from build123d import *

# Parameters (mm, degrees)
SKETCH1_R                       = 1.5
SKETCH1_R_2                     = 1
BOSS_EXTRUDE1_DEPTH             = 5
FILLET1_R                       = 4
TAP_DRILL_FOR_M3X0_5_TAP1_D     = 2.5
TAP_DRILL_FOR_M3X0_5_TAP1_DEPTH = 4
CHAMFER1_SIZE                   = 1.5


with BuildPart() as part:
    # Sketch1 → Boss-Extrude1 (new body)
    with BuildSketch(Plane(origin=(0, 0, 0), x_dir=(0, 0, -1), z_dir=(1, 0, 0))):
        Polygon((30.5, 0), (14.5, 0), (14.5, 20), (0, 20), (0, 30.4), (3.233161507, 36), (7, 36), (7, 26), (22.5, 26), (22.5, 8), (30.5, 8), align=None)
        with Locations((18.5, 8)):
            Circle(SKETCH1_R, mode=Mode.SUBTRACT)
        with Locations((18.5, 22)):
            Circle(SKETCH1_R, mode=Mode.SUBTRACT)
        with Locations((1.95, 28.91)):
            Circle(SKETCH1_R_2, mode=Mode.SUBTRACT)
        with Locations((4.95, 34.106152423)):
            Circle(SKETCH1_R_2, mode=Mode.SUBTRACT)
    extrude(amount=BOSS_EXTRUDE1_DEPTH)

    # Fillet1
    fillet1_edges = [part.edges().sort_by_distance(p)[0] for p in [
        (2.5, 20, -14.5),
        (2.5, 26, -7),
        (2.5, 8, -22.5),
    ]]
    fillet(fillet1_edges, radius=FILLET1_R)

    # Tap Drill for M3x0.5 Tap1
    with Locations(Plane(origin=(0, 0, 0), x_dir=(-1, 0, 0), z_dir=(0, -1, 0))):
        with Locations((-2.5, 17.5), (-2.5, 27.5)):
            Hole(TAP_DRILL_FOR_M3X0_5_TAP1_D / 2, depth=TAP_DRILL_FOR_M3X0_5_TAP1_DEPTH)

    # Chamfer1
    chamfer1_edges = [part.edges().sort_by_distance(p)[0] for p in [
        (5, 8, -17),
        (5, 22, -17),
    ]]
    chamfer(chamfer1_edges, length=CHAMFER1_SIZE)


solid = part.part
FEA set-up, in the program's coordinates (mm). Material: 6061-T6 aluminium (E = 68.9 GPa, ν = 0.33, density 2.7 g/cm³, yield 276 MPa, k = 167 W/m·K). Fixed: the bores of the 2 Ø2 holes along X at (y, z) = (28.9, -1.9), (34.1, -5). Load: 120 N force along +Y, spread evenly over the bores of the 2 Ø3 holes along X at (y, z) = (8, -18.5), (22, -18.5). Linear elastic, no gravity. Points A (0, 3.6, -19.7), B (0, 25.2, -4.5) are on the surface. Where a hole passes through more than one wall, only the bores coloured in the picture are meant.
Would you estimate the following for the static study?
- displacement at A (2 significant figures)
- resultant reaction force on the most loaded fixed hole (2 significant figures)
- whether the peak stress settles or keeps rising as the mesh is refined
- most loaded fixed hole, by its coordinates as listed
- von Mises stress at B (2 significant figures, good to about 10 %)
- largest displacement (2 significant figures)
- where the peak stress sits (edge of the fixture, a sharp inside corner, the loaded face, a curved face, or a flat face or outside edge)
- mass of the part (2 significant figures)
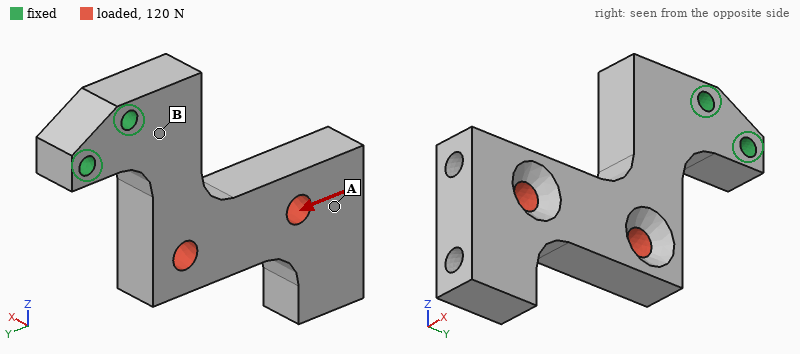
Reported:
58 µm
300 N
keeps rising
(34.1, -5)
15 MPa
79 µm
edge of the fixture
5.4 g
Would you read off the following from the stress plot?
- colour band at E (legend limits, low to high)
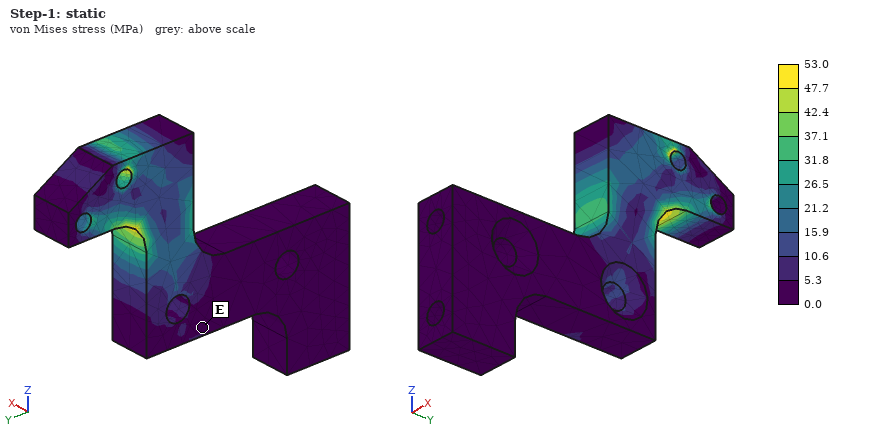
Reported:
0.0 to 5.3 MPa
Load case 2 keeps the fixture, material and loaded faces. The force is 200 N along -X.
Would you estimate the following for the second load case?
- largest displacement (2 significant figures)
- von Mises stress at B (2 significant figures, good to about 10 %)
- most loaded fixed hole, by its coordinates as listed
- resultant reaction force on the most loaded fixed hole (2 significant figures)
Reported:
0.36 mm
100 MPa
(28.9, -1.9)
210 N
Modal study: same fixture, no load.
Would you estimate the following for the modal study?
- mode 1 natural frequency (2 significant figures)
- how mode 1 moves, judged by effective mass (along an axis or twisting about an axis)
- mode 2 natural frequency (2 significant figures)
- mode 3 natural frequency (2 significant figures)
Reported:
2200 Hz
along X
2900 Hz
8200 Hz
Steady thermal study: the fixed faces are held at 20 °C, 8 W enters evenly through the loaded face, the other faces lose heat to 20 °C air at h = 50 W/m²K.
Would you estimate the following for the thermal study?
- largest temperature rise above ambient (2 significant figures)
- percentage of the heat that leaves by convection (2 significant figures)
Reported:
27 K
16 %
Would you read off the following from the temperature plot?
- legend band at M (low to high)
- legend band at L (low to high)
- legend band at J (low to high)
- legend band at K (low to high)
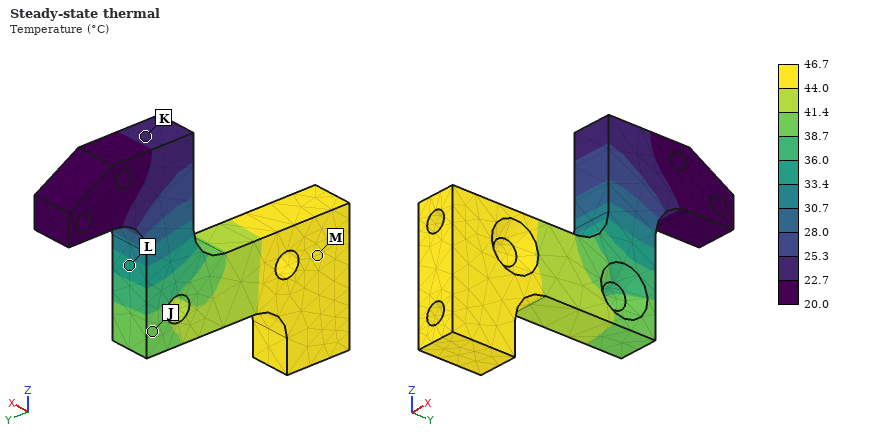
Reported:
44.0 to 46.7 °C
33.4 to 36.0 °C
38.7 to 41.4 °C
22.7 to 25.3 °C
